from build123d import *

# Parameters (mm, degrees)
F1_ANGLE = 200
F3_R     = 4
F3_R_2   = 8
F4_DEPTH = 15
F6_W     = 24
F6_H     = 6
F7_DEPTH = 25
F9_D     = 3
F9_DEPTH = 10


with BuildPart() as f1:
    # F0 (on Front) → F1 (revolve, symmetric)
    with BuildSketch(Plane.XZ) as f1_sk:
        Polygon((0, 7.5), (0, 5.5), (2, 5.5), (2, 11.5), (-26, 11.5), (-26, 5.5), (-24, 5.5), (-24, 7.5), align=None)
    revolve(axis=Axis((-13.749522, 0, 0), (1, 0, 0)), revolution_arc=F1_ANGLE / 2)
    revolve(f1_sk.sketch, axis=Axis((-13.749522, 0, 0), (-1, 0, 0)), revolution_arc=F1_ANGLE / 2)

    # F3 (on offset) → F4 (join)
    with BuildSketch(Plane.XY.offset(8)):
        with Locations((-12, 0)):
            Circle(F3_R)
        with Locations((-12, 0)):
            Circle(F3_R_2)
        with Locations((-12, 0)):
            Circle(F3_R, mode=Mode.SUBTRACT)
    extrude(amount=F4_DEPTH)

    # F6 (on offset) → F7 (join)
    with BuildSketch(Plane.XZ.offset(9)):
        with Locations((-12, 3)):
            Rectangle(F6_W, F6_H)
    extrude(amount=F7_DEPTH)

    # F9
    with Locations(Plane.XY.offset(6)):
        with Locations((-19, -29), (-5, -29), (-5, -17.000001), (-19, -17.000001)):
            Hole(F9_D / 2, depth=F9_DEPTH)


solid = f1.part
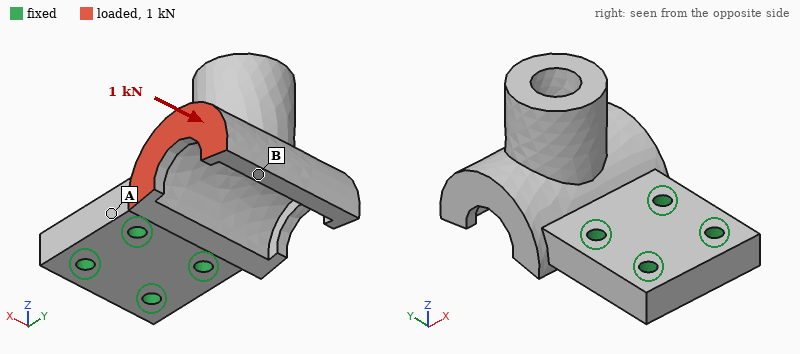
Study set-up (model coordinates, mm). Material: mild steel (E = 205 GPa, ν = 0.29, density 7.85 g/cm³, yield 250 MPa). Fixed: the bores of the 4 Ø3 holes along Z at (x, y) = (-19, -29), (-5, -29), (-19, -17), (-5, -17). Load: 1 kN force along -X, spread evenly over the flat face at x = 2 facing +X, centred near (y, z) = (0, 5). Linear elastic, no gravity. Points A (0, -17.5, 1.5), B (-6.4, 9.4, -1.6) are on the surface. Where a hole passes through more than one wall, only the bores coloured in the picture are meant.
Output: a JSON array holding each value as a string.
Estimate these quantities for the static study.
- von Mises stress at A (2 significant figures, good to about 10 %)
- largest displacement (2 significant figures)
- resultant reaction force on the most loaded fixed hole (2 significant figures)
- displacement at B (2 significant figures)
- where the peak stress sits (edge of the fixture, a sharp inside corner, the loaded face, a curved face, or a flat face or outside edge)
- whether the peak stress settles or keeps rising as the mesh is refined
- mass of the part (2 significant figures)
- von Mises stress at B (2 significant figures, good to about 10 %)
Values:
["22 MPa", "14 µm", "1.0 kN", "12 µm", "edge of the fixture", "keeps rising", "70 g", "10 MPa"]
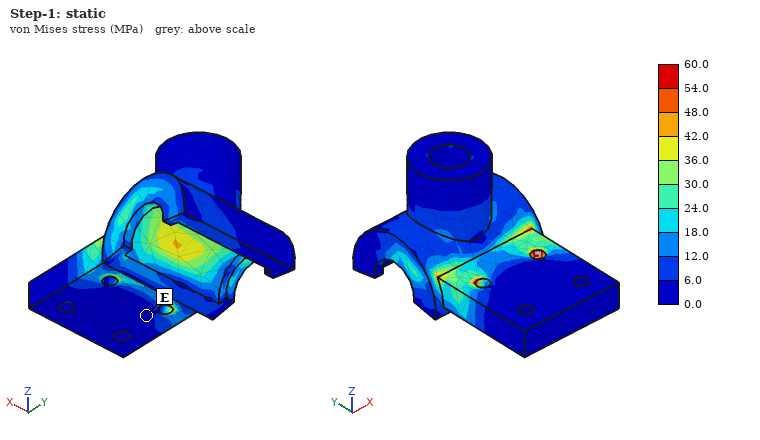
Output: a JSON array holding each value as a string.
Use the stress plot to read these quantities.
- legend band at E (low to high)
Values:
["0.0 to 6.0 MPa"]
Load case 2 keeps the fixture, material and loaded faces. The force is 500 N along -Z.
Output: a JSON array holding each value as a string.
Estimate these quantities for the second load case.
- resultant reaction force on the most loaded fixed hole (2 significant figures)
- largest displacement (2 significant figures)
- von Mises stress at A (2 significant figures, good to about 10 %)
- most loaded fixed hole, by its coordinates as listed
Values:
["730 N", "40 µm", "21 MPa", "(-5, -17)"]
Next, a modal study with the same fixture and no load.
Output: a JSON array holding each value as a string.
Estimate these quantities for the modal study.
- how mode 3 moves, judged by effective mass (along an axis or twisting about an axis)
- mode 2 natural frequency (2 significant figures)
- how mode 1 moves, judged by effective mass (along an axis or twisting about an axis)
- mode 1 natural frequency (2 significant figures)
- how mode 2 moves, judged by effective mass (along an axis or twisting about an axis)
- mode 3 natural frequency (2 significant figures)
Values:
["along X", "7900 Hz", "along Z", "3400 Hz", "twisting about Y", "10 kHz"]
